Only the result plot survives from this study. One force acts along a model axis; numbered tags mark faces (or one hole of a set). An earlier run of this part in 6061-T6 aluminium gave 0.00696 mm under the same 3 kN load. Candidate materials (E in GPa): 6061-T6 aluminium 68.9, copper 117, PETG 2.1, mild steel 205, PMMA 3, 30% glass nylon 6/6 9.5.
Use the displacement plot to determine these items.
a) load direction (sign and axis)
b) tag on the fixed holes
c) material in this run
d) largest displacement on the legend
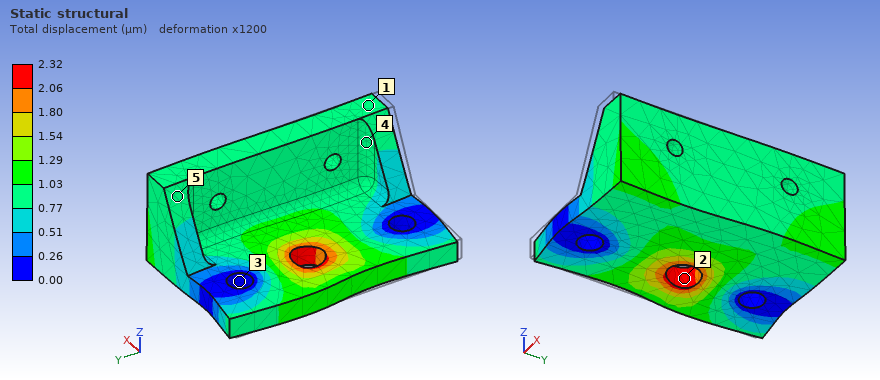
+Y
3
mild steel
2.32 µm
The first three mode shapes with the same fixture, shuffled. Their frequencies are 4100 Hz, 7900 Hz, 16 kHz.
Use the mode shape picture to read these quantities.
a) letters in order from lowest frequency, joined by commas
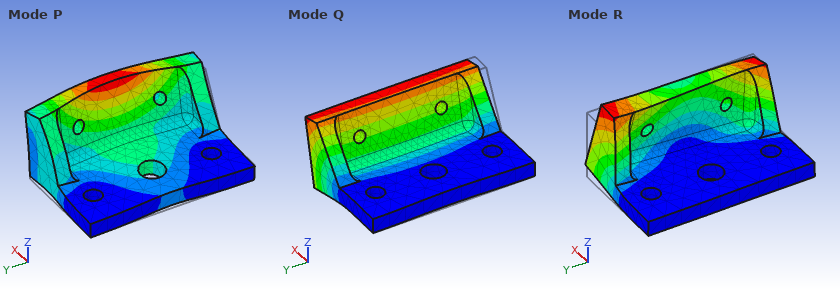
Q, R, P
